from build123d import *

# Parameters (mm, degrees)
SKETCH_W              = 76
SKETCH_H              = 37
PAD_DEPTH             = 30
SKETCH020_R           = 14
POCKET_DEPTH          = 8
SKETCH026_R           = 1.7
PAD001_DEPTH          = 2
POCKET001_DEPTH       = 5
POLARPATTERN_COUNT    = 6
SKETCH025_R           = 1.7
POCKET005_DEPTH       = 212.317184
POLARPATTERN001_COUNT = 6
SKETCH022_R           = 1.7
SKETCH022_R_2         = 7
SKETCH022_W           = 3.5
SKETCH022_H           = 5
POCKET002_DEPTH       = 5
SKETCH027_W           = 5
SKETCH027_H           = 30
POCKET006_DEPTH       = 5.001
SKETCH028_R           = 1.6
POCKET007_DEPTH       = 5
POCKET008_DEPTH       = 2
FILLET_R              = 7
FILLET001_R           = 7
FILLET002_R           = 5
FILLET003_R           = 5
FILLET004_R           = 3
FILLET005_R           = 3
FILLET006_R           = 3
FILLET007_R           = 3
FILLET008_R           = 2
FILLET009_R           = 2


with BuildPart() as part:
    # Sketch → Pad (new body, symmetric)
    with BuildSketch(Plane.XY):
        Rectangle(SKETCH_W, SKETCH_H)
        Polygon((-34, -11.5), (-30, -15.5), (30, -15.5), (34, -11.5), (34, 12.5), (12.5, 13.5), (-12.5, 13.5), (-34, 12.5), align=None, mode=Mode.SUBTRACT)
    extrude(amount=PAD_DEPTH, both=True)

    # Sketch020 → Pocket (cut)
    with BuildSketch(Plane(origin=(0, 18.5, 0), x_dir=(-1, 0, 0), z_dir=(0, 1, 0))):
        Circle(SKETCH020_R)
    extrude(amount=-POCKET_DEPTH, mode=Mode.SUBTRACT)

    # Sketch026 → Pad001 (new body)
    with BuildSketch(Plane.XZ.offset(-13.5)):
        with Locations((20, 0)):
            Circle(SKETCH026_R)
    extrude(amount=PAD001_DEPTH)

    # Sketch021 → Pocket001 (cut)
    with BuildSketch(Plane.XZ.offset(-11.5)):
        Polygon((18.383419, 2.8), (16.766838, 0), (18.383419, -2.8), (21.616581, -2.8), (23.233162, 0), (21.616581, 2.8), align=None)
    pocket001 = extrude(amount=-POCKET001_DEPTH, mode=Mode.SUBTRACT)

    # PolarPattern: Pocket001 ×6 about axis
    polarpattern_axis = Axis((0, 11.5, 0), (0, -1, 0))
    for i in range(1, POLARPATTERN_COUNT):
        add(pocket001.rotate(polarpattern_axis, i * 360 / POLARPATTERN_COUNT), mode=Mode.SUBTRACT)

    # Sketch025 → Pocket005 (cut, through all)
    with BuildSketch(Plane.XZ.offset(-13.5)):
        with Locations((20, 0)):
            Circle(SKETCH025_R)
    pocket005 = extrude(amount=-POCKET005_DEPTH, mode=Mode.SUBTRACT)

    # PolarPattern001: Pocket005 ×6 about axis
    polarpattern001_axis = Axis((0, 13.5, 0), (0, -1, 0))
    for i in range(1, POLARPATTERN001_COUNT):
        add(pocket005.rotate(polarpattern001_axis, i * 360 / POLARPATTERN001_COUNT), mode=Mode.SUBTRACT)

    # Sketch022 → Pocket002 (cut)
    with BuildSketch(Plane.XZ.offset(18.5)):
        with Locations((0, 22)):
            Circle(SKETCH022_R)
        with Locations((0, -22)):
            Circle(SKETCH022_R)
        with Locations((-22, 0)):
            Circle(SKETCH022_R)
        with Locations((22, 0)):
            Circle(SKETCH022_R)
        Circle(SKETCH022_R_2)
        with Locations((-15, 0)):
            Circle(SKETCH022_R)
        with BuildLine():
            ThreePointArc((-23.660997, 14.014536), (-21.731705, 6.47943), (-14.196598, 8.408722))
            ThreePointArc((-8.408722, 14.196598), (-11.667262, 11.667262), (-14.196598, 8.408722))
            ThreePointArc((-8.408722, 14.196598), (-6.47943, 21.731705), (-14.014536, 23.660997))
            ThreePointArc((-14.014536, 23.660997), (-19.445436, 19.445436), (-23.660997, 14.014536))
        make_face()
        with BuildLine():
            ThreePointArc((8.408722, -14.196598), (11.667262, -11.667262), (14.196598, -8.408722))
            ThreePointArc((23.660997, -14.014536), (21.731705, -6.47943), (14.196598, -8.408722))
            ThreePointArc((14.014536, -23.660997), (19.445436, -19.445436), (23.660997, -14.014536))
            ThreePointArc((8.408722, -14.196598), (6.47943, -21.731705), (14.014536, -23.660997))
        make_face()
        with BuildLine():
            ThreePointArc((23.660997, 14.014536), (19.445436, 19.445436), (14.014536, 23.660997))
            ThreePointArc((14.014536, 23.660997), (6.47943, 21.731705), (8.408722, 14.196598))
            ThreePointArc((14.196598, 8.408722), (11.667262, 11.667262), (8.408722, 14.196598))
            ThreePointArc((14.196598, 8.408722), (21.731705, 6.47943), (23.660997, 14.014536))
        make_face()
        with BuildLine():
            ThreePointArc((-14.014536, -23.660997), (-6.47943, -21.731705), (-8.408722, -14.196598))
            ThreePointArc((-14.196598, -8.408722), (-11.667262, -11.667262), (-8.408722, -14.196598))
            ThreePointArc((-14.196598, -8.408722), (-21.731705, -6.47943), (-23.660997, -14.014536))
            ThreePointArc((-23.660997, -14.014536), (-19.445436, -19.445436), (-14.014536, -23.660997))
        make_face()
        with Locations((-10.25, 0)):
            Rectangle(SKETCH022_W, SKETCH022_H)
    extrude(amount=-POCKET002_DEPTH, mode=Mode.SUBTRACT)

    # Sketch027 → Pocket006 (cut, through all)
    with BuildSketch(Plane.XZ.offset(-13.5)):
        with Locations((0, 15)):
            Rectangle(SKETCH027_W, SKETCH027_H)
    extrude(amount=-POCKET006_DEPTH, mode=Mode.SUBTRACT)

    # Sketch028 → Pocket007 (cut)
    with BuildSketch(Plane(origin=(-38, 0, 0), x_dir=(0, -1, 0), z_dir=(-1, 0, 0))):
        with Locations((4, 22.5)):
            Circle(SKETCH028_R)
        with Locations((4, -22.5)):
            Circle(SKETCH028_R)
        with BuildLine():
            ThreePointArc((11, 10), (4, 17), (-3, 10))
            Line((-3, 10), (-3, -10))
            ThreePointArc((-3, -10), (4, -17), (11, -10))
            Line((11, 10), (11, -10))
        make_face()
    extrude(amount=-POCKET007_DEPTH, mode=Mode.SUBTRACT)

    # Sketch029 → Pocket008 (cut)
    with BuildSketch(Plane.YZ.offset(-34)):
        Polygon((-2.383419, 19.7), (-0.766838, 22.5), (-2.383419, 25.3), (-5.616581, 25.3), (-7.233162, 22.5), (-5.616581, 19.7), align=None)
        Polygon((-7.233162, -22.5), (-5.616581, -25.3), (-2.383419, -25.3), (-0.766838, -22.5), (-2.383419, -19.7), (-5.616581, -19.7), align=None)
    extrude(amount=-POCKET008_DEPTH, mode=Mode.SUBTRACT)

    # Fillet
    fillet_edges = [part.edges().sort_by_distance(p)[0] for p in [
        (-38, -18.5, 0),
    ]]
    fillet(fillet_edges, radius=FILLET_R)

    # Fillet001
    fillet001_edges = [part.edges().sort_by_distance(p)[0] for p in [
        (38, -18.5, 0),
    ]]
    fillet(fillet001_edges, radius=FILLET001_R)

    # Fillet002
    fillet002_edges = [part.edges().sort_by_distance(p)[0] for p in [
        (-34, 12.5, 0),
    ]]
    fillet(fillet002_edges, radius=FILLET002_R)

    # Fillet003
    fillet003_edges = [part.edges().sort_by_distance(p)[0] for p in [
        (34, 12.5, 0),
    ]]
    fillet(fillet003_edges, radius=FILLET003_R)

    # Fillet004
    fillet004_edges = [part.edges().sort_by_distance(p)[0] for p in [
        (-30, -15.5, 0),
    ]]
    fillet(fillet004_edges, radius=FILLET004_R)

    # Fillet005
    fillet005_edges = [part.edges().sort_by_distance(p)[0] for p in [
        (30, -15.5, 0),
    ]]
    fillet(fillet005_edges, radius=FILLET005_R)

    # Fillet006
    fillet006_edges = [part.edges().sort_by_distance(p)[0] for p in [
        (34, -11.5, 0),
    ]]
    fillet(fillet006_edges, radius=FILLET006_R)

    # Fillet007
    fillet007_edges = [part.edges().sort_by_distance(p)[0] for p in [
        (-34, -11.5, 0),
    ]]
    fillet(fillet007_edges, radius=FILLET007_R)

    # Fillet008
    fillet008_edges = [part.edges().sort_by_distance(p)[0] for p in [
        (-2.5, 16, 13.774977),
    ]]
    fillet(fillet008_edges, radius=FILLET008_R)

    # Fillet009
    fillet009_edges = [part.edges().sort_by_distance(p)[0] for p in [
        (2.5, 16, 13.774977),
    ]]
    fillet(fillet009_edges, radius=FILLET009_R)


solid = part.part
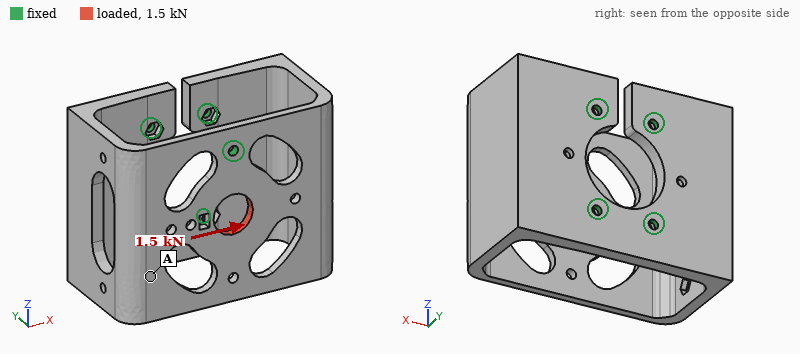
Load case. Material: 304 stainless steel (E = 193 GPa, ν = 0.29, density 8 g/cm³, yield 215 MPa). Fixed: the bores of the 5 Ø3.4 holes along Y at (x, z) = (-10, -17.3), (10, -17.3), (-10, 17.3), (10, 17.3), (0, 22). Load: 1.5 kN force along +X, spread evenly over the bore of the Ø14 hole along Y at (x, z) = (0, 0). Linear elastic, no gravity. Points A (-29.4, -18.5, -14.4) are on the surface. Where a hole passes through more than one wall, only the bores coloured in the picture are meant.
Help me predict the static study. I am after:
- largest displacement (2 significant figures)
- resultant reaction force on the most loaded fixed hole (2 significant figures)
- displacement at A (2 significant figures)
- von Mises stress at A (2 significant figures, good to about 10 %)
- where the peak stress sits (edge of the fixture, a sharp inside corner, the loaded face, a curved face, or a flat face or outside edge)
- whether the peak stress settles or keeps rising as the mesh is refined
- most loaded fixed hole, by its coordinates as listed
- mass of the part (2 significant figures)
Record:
32 µm
1.4 kN
25 µm
9.9 MPa
edge of the fixture
keeps rising
(0, 22)
340 g
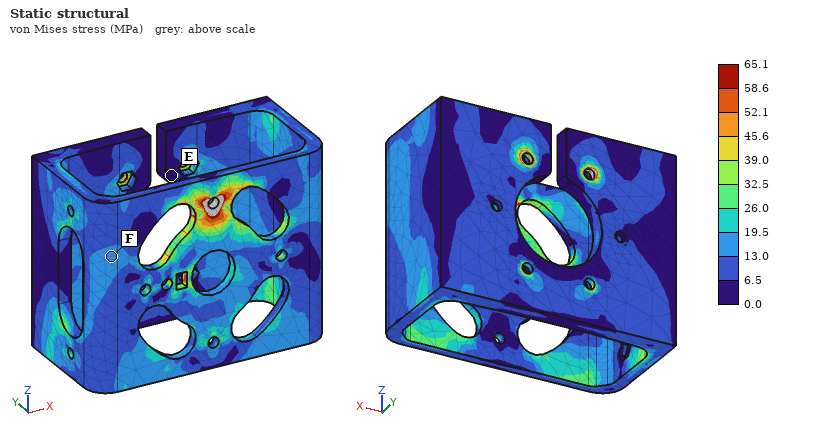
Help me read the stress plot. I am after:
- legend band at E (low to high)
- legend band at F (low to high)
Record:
0.0 to 6.5 MPa
13.0 to 19.5 MPa
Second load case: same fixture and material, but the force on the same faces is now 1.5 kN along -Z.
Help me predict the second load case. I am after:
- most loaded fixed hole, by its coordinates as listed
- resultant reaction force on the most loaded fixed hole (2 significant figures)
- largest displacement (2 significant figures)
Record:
(0, 22)
1.4 kN
7.2 µm
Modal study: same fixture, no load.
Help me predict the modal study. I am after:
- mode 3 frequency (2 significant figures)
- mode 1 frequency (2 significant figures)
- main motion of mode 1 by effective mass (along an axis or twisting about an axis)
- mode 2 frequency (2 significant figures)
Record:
3000 Hz
2100 Hz
along Y
2200 Hz
